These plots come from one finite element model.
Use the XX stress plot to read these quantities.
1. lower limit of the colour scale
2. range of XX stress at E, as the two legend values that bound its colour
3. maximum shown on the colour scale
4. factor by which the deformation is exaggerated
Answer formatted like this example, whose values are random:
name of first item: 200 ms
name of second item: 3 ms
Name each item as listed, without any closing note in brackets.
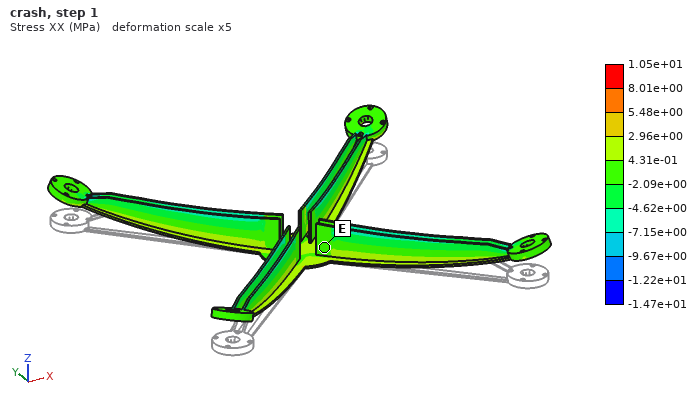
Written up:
lower limit of the colour scale: -1.47e+01 MPa
range of XX stress at E, as the two legend values that bound its colour: -2.09e+00 to 4.31e-01 MPa
maximum shown on the colour scale: 1.05e+01 MPa
factor by which the deformation is exaggerated: 5
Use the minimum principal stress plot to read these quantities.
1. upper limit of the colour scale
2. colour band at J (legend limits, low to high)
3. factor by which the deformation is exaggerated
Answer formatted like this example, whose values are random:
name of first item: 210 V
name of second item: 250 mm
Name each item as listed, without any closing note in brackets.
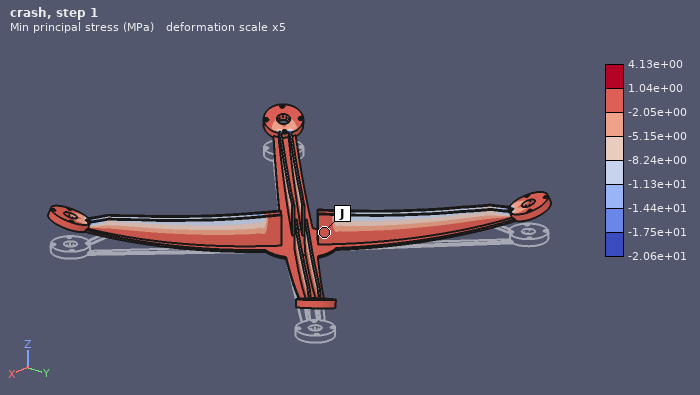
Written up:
upper limit of the colour scale: 4.13e+00 MPa
colour band at J: -2.05e+00 to 1.04e+00 MPa
factor by which the deformation is exaggerated: 5
